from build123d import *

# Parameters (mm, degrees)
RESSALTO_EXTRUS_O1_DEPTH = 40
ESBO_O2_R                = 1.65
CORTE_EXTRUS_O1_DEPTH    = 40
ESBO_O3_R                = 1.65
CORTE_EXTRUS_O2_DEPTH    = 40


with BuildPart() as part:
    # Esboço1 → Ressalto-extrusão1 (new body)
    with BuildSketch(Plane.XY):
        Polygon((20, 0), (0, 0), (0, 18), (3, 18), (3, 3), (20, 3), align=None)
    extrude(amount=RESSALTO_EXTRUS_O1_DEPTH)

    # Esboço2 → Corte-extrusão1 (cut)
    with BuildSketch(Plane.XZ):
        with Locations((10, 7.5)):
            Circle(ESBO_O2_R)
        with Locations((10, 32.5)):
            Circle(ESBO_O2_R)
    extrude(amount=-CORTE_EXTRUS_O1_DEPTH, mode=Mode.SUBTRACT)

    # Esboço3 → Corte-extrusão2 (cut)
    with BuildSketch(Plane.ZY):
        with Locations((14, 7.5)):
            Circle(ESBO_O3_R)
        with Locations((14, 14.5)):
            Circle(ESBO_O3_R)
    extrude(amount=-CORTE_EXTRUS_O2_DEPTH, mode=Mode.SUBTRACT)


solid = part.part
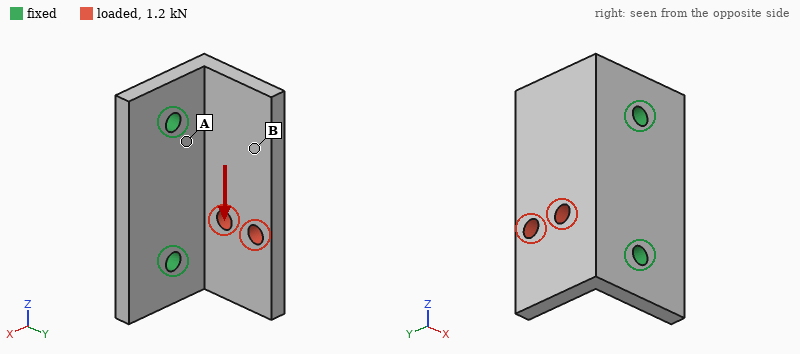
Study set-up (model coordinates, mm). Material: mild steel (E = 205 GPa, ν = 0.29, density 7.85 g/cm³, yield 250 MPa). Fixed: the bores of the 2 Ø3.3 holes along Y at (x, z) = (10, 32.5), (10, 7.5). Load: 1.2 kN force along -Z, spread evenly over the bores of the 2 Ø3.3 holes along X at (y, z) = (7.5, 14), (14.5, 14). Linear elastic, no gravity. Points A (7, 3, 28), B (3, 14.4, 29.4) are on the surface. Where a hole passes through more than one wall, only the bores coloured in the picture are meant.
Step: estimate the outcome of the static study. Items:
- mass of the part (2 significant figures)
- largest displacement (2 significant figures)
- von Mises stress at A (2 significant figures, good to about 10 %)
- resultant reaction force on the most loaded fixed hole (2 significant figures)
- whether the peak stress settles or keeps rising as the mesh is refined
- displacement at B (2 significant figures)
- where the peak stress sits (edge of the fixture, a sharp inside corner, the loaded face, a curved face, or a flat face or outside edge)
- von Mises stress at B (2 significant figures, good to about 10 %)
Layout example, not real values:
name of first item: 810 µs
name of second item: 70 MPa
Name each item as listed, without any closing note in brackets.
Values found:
mass of the part: 32 g
largest displacement: 22 µm
von Mises stress at A: 56 MPa
resultant reaction force on the most loaded fixed hole: 820 N
whether the peak stress settles or keeps rising as the mesh is refined: keeps rising
displacement at B: 13 µm
where the peak stress sits: edge of the fixture
von Mises stress at B: 22 MPa
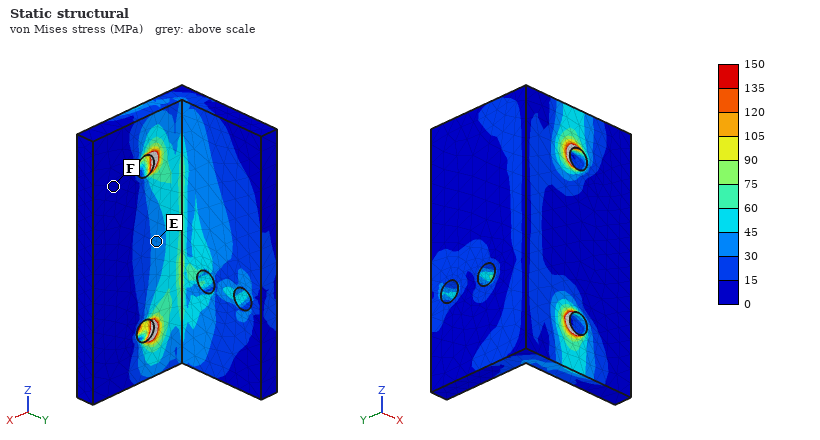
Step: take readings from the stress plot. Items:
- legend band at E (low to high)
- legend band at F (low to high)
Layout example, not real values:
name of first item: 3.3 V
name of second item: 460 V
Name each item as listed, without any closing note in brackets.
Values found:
legend band at E: 30 to 45 MPa
legend band at F: 0 to 15 MPa
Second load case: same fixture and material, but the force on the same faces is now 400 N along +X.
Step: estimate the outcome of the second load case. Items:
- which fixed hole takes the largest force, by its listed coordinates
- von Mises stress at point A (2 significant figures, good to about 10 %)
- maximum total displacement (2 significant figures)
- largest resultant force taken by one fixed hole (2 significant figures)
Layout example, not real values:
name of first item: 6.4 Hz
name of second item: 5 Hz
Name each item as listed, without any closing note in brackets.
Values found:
which fixed hole takes the largest force, by its listed coordinates: (10, 7.5)
von Mises stress at point A: 49 MPa
maximum total displacement: 51 µm
largest resultant force taken by one fixed hole: 300 N
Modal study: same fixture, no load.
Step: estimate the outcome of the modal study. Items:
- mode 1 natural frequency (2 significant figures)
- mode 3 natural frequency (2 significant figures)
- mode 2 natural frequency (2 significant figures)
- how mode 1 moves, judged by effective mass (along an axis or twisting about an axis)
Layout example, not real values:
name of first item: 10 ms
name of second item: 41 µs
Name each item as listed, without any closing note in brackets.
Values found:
mode 1 natural frequency: 5000 Hz
mode 3 natural frequency: 14 kHz
mode 2 natural frequency: 8300 Hz
how mode 1 moves, judged by effective mass: along X
